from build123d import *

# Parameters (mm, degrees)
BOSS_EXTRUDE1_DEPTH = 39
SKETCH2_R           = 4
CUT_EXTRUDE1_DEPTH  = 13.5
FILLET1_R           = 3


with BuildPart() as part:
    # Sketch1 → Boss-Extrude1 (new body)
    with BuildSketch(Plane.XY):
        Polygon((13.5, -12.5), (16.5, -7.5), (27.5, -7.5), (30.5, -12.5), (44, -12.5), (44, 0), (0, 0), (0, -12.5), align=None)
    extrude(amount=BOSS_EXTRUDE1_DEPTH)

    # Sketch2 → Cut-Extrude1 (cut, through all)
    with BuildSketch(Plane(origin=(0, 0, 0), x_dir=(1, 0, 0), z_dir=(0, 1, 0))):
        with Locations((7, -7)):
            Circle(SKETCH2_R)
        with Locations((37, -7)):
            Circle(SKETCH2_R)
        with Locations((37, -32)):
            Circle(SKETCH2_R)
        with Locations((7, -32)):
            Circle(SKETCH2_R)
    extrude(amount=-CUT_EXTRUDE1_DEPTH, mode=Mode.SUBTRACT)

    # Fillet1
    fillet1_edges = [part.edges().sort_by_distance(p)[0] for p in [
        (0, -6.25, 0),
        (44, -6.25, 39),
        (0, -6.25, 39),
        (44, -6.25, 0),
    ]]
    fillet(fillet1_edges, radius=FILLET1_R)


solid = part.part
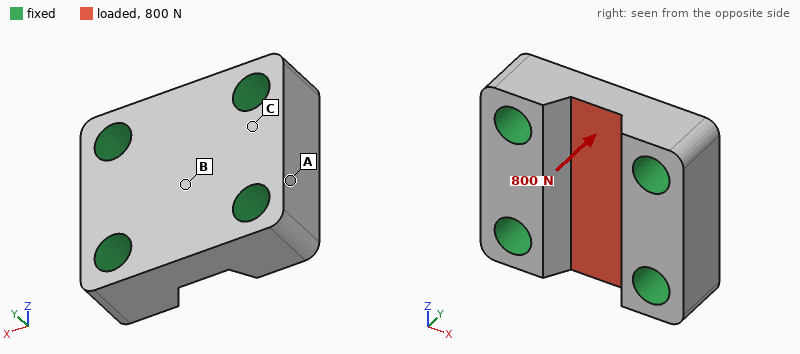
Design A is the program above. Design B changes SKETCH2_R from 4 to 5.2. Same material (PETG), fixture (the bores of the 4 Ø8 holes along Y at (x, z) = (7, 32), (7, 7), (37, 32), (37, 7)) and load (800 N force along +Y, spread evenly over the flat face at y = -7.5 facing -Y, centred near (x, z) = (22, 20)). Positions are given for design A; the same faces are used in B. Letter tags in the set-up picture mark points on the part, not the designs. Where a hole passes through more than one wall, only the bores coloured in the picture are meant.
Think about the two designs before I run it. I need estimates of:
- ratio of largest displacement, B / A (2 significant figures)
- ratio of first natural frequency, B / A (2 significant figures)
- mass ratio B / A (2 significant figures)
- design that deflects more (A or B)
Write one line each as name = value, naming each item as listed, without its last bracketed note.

ratio of largest displacement, B / A = 0.84
ratio of first natural frequency, B / A = 1.1
mass ratio B / A = 0.89
design that deflects more = A
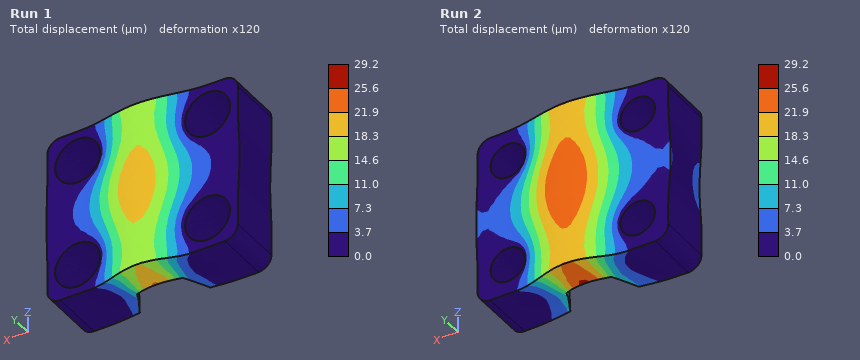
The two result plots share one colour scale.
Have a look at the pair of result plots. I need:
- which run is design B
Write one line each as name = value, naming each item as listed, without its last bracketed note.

which run is design B = Run 1
